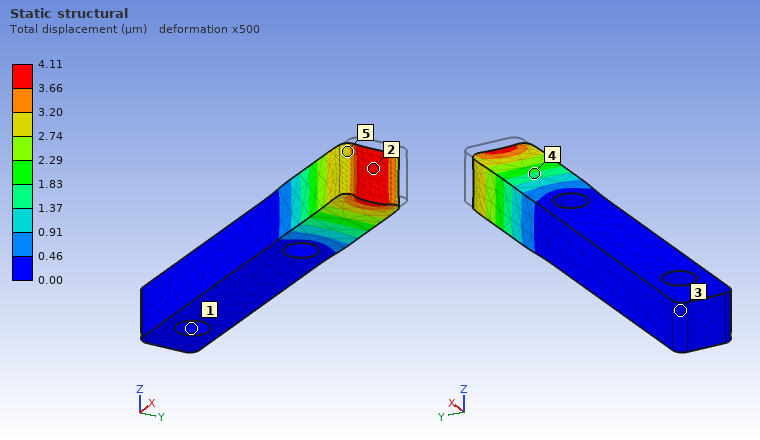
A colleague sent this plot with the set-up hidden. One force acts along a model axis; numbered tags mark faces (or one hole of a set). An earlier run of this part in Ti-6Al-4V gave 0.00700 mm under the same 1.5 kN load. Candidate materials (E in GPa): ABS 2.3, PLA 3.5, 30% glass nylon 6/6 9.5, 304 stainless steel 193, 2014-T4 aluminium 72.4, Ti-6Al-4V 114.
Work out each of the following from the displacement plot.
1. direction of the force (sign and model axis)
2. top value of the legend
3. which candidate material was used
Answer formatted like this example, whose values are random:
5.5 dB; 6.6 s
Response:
-X; 4.11 µm; 304 stainless steel
